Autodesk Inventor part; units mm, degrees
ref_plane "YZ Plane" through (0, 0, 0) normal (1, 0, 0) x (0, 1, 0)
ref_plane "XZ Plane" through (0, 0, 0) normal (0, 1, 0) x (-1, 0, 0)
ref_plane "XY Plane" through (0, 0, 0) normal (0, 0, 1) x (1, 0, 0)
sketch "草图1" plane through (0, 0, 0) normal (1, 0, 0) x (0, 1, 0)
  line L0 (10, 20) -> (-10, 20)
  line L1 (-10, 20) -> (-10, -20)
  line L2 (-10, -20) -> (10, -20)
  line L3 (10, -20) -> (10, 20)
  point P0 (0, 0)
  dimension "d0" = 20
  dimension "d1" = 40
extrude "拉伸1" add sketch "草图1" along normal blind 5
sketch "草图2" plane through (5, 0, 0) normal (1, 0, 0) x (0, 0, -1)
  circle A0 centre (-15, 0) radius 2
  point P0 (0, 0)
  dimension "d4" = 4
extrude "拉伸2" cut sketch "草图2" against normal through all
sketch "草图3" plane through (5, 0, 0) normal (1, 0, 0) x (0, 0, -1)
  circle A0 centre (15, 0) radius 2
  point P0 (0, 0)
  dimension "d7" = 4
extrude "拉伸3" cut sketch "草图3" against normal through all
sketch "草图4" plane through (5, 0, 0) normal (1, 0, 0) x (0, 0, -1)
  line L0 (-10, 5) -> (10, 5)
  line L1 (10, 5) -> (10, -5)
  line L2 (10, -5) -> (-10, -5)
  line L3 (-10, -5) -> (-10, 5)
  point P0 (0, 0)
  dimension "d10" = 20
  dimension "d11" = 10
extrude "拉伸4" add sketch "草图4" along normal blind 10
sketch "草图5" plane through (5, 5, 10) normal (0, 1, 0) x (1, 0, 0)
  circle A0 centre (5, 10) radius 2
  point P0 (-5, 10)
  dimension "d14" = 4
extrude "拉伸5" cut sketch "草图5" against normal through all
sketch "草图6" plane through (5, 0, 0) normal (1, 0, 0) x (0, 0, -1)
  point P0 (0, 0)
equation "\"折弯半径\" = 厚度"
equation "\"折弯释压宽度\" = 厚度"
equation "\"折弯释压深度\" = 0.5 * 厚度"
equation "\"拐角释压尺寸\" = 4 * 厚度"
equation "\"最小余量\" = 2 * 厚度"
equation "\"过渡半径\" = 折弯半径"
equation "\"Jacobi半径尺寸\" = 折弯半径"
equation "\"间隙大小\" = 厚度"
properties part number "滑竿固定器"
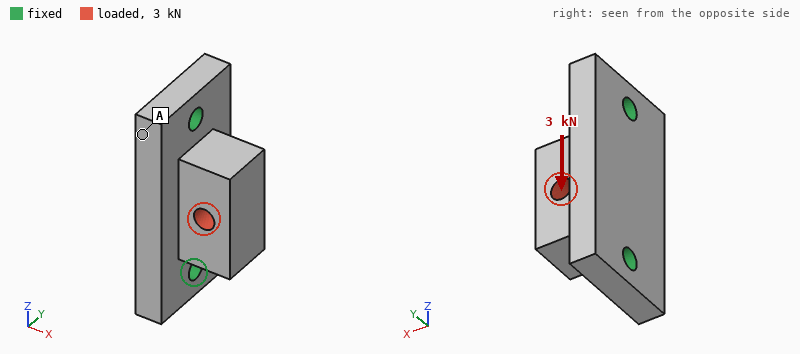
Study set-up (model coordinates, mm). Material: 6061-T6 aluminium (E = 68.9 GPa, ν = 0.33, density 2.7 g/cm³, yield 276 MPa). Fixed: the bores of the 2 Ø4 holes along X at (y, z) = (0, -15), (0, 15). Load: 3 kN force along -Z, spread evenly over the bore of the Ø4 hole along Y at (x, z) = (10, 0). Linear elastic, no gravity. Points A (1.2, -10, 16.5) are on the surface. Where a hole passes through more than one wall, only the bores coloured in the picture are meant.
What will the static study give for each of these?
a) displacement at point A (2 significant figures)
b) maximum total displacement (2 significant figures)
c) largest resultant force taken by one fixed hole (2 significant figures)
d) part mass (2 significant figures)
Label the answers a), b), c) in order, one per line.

a) 3.4 µm
b) 15 µm
c) 1.7 kN
d) 16 g
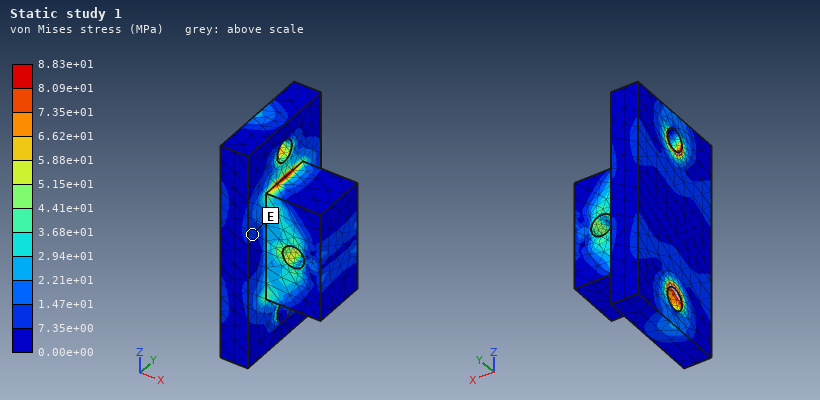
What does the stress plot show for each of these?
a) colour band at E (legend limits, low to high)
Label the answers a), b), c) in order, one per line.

a) 7.35e+00 to 1.47e+01 MPa
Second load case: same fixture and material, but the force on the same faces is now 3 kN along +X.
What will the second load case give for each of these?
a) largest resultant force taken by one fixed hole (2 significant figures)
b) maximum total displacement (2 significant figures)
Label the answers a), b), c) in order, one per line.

a) 1.6 kN
b) 17 µm
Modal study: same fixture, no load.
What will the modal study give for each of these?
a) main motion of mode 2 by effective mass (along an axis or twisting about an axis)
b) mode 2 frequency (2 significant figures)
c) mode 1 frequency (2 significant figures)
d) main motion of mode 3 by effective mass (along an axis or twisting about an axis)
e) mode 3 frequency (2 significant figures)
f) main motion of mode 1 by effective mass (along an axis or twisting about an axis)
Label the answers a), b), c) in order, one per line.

a) along X
b) 23 kHz
c) 14 kHz
d) along Y
e) 32 kHz
f) along Y
